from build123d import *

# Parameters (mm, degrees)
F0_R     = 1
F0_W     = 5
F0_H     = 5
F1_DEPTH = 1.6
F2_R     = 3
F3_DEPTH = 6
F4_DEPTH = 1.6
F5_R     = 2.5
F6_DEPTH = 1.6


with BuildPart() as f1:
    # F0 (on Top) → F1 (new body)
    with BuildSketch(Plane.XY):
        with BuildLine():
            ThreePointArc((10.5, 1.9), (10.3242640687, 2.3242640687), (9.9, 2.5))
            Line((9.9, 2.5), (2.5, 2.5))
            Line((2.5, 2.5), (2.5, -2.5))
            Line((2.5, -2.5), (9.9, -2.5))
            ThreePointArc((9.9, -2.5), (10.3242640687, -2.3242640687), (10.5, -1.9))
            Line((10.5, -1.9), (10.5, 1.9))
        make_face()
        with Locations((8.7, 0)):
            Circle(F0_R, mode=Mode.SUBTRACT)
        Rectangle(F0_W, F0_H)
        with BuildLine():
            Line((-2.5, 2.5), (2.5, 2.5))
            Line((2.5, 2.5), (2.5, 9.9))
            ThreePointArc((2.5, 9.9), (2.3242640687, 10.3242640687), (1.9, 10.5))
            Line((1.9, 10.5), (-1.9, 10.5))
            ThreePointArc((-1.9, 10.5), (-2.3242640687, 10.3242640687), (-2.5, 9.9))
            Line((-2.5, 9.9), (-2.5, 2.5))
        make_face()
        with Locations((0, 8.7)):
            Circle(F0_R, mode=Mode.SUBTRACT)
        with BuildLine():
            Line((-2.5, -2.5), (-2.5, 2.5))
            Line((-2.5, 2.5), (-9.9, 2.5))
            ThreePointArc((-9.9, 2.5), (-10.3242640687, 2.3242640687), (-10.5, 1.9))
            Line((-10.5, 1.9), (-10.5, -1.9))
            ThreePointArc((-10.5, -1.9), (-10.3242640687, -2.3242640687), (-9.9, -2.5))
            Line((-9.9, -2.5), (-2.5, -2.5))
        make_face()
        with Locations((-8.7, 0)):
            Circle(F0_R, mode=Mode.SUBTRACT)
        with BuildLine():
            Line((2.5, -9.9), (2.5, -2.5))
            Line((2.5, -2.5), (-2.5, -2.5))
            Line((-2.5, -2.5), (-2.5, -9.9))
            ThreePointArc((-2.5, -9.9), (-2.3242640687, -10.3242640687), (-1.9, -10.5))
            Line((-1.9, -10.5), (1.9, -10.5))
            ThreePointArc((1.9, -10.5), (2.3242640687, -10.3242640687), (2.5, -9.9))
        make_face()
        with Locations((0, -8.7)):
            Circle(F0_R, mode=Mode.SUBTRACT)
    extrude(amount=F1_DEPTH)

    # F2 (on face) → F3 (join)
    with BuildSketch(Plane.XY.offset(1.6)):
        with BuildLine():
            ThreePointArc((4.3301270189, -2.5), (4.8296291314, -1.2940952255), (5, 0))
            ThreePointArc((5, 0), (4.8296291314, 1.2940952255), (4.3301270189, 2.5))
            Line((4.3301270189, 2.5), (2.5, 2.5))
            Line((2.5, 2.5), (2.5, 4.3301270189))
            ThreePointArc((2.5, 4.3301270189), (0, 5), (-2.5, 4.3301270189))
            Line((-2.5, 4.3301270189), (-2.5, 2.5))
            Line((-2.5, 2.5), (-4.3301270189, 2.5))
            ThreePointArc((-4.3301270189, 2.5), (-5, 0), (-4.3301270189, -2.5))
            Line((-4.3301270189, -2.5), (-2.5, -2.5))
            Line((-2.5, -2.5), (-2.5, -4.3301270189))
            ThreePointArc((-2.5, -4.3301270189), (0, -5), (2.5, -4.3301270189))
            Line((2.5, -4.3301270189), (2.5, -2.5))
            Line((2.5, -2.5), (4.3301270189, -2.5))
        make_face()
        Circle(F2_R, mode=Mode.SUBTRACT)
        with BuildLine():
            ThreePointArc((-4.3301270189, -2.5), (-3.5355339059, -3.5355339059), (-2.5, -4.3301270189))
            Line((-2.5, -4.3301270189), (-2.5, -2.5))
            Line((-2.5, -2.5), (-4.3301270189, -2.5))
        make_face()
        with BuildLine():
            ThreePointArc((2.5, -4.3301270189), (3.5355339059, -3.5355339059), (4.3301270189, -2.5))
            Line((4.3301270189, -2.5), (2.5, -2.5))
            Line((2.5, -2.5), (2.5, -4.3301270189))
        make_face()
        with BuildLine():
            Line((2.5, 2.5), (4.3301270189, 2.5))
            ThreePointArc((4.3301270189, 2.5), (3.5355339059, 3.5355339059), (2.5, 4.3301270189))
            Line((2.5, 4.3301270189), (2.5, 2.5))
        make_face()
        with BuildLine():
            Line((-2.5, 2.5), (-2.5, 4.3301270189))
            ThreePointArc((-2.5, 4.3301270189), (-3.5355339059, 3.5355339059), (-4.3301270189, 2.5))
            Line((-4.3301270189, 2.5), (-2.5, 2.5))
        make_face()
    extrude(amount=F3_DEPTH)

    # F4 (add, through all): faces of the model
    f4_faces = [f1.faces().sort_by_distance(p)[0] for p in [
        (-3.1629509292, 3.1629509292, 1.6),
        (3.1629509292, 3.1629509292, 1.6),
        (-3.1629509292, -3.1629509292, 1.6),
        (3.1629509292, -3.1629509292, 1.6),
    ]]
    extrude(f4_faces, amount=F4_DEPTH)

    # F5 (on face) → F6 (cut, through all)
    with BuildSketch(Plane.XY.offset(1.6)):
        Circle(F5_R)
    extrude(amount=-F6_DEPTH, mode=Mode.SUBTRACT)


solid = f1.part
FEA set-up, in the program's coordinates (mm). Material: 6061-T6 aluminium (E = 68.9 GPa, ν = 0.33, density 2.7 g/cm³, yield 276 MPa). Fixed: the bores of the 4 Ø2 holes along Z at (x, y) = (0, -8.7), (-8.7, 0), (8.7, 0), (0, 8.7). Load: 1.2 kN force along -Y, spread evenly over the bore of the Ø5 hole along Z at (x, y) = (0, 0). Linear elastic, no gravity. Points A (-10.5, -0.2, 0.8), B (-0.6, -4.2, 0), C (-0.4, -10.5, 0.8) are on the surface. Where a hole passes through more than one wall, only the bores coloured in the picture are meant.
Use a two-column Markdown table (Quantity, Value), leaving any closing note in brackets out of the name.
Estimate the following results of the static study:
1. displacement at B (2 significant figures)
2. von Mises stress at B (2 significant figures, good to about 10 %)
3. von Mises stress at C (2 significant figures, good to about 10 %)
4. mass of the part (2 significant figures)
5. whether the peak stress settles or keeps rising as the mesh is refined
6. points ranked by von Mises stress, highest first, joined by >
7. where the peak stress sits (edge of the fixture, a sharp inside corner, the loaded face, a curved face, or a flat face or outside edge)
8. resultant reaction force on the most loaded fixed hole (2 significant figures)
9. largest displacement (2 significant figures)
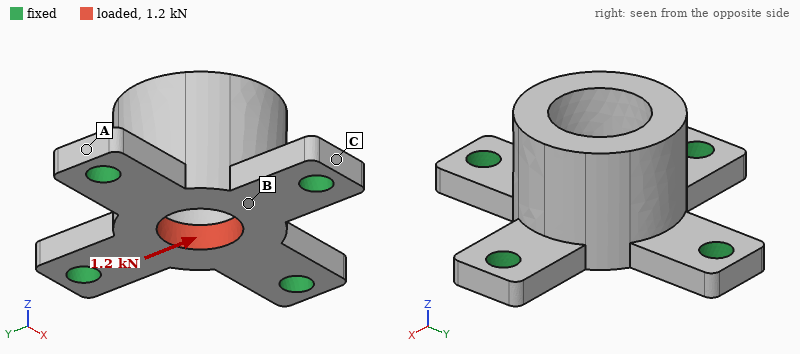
| Quantity | Value |
|---|---|
| displacement at B | 3.8 µm |
| von Mises stress at B | 65 MPa |
| von Mises stress at C | 28 MPa |
| mass of the part | 1.5 g |
| whether the peak stress settles or keeps rising as the mesh is refined | keeps rising |
| points ranked by von Mises stress, highest first, joined by > | B > C > A |
| where the peak stress sits | edge of the fixture |
| resultant reaction force on the most loaded fixed hole | 500 N |
| largest displacement | 7.3 µm |
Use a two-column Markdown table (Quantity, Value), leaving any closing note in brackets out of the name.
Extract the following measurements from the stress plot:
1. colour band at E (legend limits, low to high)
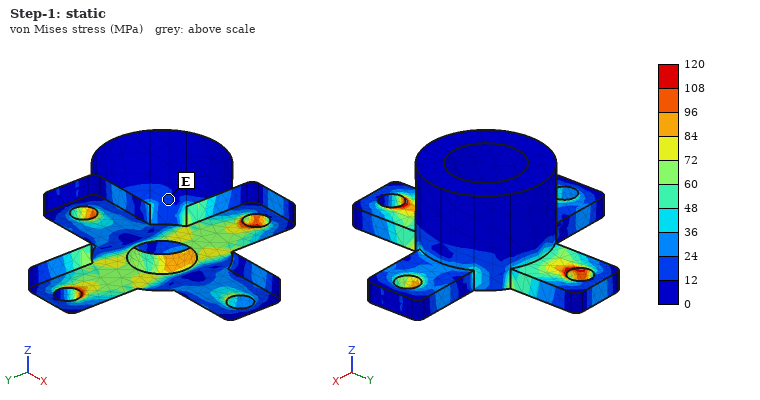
| Quantity | Value |
|---|---|
| colour band at E | 12 to 24 MPa |
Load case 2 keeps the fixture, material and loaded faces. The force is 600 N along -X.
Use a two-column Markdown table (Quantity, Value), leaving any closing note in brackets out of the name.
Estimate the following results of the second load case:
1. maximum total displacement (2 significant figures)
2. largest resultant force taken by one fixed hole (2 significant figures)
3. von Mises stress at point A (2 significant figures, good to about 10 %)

| Quantity | Value |
|---|---|
| maximum total displacement | 3.6 µm |
| largest resultant force taken by one fixed hole | 250 N |
| von Mises stress at point A | 14 MPa |
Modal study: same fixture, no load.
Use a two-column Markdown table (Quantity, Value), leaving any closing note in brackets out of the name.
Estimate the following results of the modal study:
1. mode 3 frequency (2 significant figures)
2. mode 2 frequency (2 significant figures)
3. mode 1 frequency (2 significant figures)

| Quantity | Value |
|---|---|
| mode 3 frequency | 35 kHz |
| mode 2 frequency | 34 kHz |
| mode 1 frequency | 34 kHz |
